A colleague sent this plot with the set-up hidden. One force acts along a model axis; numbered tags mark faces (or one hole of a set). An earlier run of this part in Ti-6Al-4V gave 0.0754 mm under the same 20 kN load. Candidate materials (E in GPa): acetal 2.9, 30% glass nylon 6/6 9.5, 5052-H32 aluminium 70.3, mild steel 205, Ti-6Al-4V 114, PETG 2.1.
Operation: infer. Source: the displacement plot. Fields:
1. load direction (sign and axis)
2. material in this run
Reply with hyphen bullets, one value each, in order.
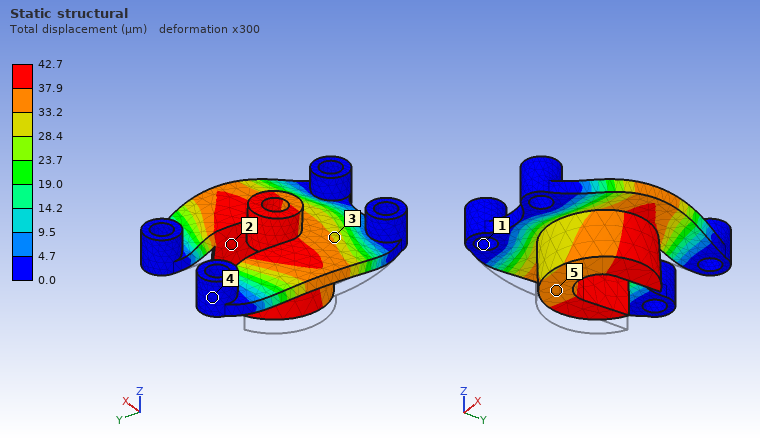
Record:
- +Z
- mild steel
